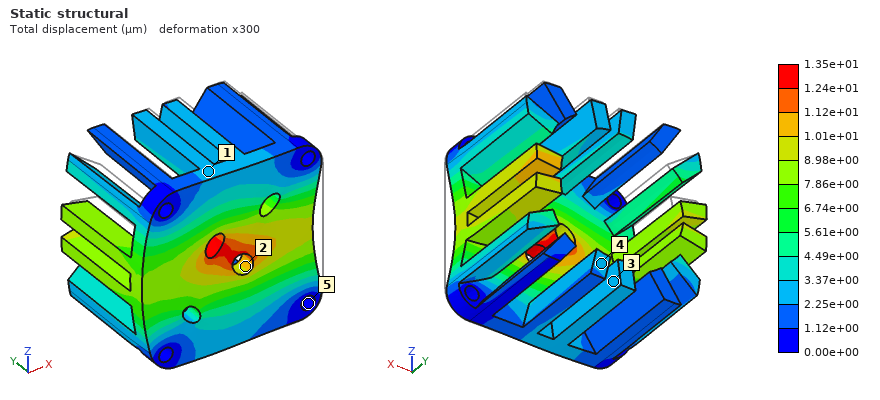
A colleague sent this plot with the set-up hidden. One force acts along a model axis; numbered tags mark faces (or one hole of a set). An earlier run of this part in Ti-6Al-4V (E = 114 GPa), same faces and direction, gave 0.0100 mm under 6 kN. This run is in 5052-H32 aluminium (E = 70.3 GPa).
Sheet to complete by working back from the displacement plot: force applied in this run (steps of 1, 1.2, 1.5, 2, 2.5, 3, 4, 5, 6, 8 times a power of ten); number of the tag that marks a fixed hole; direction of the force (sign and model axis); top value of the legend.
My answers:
5 kN
5
-X
1.35e+01 µm
